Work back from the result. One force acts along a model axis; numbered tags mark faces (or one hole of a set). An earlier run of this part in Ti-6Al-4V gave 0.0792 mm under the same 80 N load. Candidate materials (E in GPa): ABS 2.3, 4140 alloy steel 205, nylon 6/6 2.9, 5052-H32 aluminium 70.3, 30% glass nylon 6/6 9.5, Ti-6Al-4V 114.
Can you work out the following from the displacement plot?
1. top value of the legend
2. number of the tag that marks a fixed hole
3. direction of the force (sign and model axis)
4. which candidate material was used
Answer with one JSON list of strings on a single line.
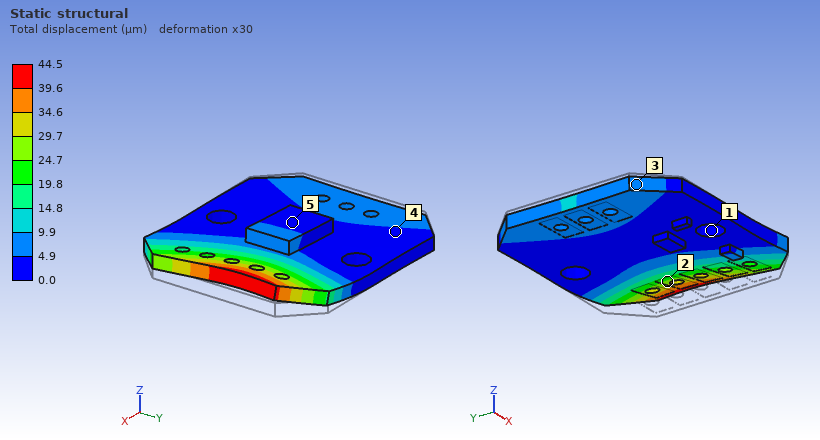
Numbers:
["44.5 µm", "1", "+Z", "4140 alloy steel"]
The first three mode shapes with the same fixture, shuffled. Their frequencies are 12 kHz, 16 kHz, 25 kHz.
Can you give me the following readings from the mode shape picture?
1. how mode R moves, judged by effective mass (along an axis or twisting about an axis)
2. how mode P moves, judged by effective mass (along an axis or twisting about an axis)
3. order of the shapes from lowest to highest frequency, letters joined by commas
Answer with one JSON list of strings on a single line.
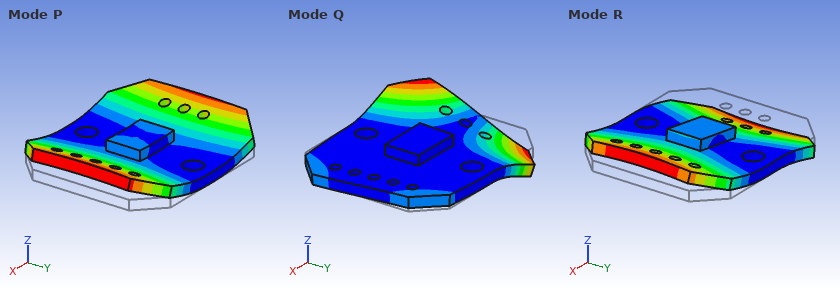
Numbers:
["twisting about Y", "along Z", "R, P, Q"]
